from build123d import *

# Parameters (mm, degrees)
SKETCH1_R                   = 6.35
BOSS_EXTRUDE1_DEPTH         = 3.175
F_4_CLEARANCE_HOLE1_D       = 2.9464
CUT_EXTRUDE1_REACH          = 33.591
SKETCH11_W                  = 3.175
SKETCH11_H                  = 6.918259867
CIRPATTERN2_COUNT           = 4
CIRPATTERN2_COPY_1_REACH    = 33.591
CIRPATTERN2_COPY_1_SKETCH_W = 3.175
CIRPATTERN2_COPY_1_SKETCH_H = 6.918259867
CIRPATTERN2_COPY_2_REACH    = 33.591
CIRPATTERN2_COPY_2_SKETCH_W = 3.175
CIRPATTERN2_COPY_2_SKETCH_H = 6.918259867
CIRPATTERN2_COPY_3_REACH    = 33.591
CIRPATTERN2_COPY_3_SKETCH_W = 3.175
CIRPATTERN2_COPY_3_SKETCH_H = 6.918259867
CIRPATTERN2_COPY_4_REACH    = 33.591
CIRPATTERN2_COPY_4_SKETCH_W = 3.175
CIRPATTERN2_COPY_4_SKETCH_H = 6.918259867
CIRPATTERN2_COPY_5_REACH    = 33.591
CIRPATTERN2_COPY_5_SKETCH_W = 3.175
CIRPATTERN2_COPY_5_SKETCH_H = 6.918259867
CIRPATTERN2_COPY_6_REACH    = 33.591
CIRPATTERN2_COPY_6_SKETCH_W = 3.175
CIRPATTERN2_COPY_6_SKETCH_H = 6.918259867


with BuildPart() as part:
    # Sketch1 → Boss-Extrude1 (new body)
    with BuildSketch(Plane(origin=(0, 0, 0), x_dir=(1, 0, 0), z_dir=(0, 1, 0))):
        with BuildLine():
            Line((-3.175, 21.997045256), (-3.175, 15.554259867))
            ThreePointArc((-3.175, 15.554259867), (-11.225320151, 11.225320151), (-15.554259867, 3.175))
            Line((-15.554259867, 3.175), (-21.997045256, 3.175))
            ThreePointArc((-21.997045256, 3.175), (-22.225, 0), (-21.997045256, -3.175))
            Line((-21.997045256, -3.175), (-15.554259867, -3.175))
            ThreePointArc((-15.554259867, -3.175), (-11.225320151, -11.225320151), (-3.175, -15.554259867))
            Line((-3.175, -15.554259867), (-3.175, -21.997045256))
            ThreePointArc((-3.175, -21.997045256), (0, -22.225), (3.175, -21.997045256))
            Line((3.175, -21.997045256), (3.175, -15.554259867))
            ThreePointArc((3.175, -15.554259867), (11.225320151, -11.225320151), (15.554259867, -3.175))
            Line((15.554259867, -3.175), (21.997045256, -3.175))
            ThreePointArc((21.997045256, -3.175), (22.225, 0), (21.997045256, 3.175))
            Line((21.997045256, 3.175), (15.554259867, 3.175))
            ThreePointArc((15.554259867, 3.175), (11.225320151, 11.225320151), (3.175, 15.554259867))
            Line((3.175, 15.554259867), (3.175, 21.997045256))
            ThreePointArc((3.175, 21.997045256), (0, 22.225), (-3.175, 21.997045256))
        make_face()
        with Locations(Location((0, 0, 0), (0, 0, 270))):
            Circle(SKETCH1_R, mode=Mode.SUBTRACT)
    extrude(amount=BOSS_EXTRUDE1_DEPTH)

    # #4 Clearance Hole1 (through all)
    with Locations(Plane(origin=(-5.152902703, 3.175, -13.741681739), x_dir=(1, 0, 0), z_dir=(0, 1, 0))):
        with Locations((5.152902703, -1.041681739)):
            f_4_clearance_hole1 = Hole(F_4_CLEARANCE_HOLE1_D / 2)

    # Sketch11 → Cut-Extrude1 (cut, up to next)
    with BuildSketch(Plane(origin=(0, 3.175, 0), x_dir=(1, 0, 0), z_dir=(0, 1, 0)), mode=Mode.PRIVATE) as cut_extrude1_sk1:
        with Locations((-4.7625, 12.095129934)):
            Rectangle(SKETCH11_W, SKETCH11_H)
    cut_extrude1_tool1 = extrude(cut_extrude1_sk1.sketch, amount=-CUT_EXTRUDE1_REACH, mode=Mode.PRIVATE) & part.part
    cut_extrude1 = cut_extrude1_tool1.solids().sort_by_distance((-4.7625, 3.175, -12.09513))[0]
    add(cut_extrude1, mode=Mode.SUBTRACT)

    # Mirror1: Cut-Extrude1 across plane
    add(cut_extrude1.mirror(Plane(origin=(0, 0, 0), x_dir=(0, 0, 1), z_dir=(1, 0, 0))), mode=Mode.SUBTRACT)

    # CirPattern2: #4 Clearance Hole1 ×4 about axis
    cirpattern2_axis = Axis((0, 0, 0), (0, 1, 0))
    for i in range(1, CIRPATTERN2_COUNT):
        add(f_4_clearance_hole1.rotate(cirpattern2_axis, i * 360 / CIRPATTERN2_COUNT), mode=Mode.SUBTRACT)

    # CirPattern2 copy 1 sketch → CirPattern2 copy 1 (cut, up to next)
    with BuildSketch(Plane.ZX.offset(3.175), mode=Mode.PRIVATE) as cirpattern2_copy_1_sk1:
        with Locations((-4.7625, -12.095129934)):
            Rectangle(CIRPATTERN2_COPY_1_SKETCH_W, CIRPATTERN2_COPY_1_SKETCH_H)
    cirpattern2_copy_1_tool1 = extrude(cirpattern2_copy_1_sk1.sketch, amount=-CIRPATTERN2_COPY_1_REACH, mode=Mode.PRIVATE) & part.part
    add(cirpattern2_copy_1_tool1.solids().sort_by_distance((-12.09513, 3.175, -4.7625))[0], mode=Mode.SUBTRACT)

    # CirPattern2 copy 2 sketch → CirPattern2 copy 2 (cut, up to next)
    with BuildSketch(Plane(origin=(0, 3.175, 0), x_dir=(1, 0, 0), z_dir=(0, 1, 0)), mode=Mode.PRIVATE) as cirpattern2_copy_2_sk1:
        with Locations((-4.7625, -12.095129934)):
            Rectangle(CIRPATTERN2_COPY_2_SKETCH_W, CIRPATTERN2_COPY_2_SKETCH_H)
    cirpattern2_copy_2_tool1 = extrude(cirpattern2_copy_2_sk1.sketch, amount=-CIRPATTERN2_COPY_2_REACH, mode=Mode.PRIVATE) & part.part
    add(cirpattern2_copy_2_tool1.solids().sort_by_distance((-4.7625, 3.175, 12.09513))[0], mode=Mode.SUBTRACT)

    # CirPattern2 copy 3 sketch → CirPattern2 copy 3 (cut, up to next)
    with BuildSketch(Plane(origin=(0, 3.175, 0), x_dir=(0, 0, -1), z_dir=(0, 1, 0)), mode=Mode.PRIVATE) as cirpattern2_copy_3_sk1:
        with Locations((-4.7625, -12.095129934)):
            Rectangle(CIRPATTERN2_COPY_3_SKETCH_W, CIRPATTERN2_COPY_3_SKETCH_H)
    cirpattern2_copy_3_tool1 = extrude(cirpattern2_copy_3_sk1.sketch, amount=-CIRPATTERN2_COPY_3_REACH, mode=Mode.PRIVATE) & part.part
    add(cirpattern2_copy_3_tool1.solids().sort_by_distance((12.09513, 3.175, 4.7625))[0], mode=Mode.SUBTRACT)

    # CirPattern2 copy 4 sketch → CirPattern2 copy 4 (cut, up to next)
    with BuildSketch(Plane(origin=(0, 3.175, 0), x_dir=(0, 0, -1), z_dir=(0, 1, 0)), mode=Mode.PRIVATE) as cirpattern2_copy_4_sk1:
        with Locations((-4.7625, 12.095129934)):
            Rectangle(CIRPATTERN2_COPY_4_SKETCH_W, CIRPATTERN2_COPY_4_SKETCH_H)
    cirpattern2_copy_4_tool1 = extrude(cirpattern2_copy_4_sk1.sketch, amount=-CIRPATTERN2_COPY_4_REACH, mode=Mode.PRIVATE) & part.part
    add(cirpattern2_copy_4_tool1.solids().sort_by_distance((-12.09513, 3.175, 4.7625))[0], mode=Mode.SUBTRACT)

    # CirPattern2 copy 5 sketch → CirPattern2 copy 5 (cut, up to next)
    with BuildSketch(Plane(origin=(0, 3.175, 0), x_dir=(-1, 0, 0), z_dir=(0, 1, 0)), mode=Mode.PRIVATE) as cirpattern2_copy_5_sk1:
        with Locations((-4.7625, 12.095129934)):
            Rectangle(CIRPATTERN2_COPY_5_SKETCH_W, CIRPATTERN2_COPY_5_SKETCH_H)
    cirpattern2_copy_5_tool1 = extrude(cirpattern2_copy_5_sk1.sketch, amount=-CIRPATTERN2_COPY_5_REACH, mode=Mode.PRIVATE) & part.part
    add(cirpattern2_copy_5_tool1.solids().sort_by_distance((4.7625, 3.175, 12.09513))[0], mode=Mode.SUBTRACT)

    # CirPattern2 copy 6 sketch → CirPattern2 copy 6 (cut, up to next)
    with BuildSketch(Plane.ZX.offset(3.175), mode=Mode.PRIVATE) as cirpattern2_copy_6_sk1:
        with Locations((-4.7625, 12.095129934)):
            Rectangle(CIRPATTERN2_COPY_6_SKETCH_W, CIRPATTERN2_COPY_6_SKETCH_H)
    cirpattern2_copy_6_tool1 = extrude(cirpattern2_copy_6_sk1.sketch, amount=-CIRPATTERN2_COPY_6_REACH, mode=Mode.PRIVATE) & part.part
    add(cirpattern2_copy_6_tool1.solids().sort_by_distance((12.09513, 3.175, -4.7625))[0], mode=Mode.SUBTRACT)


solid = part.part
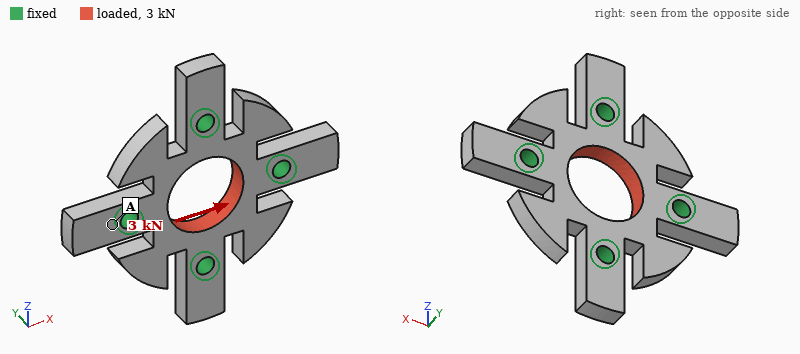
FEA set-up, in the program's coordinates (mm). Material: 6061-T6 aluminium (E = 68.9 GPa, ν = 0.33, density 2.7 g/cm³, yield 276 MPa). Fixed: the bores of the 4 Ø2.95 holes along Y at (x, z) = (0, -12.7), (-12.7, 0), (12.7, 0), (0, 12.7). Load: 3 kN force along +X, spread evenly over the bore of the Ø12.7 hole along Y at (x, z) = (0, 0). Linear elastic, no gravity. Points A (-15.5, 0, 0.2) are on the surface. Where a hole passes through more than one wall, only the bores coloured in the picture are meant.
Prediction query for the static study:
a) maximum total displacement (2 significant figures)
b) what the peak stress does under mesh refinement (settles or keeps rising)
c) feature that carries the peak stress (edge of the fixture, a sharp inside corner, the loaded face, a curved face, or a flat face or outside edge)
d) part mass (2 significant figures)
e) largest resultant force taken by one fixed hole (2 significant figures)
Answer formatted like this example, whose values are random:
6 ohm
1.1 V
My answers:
16 µm
keeps rising
edge of the fixture
5.4 g
980 N
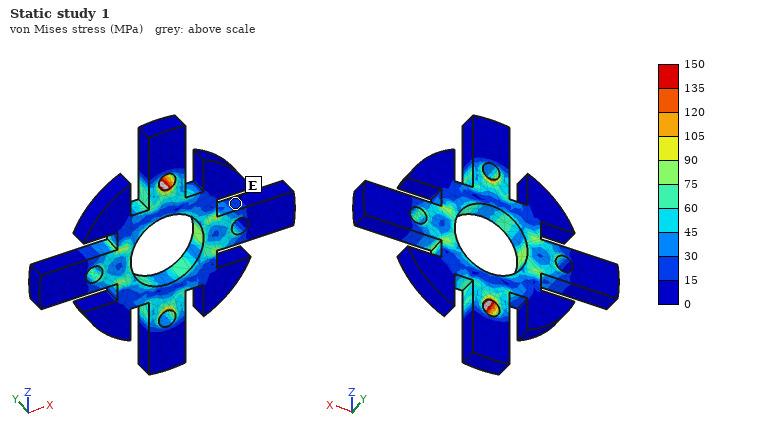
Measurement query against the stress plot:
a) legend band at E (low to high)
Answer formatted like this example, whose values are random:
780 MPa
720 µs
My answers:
15 to 30 MPa
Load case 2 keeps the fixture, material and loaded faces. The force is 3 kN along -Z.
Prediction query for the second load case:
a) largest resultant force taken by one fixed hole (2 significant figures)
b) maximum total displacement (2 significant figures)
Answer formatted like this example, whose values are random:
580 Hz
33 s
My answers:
980 N
16 µm
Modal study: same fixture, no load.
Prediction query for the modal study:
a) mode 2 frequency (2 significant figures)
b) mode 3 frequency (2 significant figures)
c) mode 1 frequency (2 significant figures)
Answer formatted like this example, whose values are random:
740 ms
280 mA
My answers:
15 kHz
15 kHz
14 kHz
